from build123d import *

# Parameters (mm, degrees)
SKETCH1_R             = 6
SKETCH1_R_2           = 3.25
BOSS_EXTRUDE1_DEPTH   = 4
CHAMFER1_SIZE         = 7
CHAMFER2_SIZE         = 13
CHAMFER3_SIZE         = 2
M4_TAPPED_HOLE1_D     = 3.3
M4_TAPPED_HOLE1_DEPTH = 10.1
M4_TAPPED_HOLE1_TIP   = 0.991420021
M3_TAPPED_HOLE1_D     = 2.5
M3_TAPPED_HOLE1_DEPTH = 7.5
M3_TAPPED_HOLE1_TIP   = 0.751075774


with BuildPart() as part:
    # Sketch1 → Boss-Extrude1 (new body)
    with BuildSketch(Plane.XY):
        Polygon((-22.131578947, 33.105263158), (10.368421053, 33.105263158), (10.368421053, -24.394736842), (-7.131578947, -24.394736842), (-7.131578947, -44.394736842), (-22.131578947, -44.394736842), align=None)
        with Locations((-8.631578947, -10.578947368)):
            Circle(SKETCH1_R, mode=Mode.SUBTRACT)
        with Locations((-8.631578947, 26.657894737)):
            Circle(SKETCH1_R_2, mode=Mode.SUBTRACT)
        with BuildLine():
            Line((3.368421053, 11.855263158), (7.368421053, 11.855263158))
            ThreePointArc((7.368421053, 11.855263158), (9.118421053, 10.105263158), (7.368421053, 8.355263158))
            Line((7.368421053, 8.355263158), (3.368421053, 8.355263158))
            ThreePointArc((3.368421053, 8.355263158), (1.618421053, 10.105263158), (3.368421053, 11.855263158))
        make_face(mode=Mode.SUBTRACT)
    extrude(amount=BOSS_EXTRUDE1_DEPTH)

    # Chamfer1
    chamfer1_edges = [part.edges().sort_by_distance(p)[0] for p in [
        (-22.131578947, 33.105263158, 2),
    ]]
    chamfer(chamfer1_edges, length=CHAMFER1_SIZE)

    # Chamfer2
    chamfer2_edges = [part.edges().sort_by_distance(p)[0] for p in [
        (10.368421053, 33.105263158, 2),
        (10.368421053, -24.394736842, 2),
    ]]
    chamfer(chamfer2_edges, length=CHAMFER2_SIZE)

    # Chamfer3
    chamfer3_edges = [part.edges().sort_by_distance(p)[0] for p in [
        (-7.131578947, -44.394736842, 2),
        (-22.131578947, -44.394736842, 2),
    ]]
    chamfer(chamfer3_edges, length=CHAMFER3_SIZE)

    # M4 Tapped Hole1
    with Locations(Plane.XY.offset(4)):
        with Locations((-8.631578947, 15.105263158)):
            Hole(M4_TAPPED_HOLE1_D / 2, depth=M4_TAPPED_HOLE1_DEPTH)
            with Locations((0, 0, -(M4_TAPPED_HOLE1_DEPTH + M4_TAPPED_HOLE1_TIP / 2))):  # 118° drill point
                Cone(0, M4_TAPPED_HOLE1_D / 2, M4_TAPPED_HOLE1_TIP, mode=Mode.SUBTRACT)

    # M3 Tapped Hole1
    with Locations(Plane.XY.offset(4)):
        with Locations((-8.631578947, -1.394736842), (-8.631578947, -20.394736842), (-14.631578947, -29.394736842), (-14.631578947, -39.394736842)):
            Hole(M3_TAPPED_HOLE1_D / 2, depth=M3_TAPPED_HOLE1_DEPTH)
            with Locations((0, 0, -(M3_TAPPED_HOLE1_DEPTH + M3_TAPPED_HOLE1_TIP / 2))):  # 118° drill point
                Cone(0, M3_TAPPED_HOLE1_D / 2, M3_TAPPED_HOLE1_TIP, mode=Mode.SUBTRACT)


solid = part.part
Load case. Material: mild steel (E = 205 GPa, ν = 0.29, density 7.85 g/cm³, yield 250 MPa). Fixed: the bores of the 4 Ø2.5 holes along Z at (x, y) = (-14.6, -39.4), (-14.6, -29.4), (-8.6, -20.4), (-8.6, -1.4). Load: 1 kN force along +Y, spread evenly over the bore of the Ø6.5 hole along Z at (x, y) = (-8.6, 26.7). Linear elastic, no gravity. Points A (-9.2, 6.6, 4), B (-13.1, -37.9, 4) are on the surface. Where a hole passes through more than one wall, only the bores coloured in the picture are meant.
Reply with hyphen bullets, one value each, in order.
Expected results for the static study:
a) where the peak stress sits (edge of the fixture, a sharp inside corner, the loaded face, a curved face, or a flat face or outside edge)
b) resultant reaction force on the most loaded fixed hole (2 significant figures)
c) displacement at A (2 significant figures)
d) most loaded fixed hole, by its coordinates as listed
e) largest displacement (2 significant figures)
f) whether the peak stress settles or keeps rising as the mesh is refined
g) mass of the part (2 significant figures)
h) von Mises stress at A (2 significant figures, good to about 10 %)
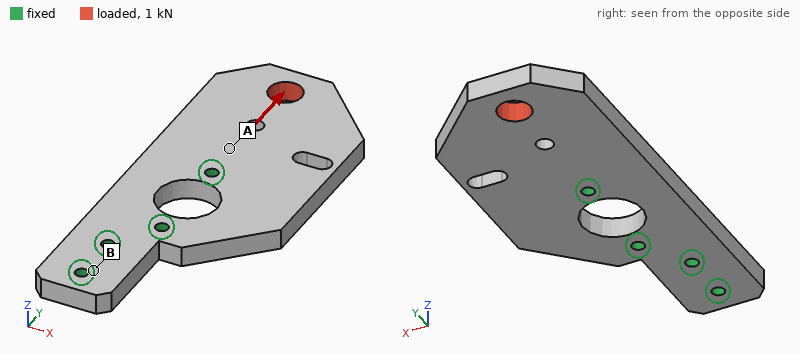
- edge of the fixture
- 740 N
- 0.68 µm
- (-8.6, -1.4)
- 2.9 µm
- keeps rising
- 56 g
- 14 MPa
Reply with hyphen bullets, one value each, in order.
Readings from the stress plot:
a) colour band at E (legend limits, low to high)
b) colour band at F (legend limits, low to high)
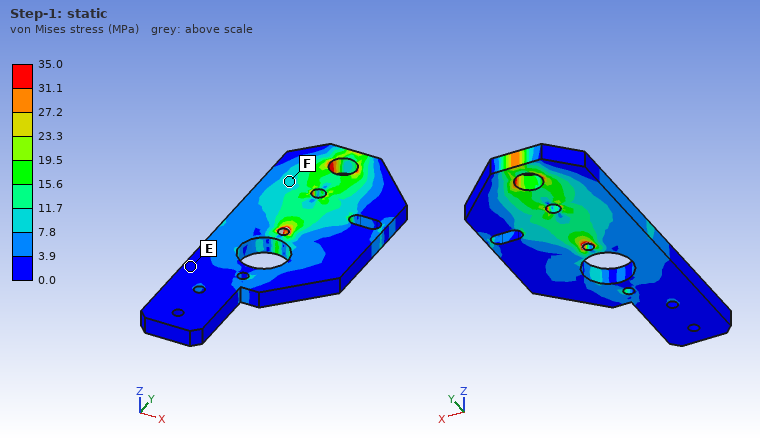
- 0.0 to 3.9 MPa
- 7.8 to 11.7 MPa
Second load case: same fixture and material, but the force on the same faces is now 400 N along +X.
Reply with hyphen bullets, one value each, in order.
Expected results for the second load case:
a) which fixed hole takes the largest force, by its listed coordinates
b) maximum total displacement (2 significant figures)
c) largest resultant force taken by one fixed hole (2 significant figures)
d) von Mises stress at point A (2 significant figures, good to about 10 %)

- (-8.6, -1.4)
- 9.4 µm
- 770 N
- 7.1 MPa
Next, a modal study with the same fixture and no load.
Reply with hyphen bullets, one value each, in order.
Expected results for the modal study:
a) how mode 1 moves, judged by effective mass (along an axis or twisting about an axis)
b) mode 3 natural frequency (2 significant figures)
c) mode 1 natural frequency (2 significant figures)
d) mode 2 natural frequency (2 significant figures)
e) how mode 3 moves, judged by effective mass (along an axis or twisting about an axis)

- along Z
- 9600 Hz
- 2900 Hz
- 5200 Hz
- along X
